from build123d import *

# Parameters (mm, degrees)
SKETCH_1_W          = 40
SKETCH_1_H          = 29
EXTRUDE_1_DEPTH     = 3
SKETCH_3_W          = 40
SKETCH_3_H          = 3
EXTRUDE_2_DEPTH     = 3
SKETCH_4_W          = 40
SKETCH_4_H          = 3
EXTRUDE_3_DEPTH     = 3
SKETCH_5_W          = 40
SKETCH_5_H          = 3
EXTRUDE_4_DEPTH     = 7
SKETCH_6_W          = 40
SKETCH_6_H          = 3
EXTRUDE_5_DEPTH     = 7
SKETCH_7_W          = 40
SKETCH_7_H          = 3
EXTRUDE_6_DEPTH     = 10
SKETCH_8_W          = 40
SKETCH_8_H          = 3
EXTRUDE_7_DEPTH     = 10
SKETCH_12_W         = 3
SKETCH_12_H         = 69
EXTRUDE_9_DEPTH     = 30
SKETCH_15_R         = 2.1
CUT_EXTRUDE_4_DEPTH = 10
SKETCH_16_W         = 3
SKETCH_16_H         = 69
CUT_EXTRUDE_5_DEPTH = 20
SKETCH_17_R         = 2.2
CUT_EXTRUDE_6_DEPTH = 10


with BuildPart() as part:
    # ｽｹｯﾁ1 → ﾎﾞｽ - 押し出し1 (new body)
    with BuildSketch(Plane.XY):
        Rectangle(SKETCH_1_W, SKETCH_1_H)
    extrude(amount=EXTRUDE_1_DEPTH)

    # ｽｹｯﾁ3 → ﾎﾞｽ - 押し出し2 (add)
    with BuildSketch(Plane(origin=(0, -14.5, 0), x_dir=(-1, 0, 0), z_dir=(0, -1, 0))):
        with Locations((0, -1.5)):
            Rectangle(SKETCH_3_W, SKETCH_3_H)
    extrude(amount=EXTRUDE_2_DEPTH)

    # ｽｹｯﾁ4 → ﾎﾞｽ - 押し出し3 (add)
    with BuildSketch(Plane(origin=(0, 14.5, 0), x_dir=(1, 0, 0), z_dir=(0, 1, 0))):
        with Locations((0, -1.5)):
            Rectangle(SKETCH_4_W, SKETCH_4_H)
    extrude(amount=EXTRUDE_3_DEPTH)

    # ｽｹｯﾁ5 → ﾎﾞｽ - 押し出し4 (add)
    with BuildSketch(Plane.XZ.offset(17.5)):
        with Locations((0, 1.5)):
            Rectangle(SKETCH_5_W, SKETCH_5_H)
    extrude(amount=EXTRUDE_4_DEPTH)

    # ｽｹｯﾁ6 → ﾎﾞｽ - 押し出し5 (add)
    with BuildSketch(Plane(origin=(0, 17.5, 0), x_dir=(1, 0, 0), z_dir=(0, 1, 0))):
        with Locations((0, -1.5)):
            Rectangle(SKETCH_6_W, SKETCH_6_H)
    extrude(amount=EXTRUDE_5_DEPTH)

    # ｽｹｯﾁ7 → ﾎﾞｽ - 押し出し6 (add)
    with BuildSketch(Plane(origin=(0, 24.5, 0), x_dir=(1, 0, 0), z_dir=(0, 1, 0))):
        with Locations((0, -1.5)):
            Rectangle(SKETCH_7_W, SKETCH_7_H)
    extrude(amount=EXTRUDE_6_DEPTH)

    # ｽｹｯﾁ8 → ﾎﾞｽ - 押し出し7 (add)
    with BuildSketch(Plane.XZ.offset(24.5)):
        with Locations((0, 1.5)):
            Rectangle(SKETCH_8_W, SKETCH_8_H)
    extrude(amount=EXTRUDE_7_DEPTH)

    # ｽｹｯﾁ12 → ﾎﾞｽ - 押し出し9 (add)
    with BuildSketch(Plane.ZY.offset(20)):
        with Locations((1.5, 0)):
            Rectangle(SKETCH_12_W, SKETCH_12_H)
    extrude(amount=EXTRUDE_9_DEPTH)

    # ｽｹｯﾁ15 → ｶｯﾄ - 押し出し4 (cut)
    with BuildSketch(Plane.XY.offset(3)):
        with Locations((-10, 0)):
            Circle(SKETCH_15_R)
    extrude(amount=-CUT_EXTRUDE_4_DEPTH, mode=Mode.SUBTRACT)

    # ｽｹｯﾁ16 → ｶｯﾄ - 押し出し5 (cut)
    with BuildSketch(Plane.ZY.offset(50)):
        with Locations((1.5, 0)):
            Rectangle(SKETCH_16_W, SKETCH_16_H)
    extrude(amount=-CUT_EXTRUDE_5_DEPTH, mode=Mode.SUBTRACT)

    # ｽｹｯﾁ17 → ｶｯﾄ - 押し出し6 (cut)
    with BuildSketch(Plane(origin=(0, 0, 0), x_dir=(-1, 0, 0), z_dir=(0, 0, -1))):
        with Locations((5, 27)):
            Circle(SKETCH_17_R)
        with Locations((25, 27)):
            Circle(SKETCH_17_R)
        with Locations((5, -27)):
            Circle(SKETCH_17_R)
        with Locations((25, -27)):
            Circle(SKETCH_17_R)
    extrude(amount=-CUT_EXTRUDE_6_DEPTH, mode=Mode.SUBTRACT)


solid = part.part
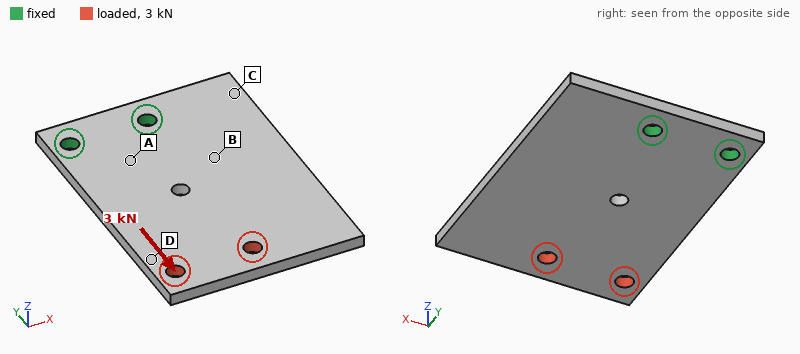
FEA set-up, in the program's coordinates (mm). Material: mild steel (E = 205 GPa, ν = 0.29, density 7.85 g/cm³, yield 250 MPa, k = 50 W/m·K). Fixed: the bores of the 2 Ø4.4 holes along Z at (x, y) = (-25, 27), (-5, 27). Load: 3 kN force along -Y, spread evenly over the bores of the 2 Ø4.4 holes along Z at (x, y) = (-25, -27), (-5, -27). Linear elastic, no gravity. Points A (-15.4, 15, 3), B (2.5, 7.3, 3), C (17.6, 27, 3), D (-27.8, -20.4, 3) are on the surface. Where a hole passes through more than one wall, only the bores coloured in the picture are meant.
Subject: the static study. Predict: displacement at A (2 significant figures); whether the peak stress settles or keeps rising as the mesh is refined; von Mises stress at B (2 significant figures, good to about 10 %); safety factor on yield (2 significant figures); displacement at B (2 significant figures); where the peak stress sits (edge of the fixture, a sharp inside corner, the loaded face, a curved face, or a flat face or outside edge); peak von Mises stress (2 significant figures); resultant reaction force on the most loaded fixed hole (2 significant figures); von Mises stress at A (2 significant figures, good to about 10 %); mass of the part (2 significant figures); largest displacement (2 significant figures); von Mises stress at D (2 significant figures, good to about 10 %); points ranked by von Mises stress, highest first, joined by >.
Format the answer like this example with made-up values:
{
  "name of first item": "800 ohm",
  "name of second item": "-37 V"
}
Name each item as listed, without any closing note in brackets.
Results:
{
  "displacement at A": "2.1 µm",
  "whether the peak stress settles or keeps rising as the mesh is refined": "settles",
  "von Mises stress at B": "15 MPa",
  "safety factor on yield": "2.5",
  "displacement at B": "2.3 µm",
  "where the peak stress sits": "the loaded face",
  "peak von Mises stress": "100 MPa",
  "resultant reaction force on the most loaded fixed hole": "1.5 kN",
  "von Mises stress at A": "26 MPa",
  "mass of the part": "79 g",
  "largest displacement": "13 µm",
  "von Mises stress at D": "45 MPa",
  "points ranked by von Mises stress, highest first, joined by >": "D > A > B > C"
}
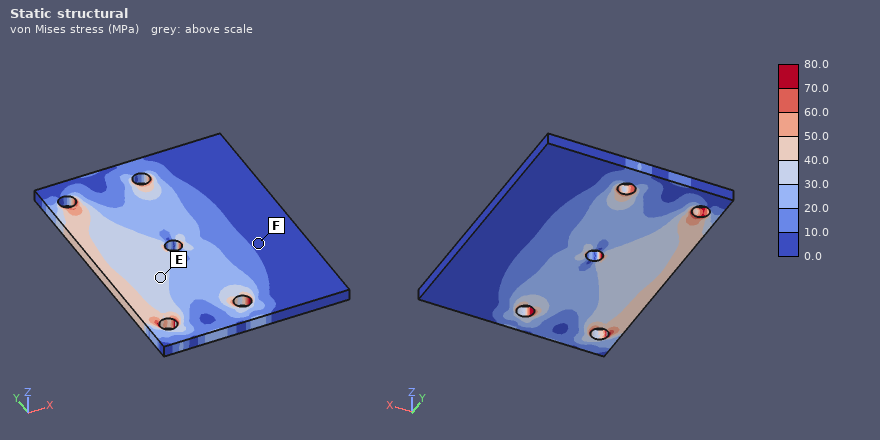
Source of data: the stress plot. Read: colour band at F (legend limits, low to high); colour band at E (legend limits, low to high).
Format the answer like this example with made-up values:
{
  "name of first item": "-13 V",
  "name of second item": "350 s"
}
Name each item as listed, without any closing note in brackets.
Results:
{
  "colour band at F": "0.0 to 10.0 MPa",
  "colour band at E": "30.0 to 40.0 MPa"
}
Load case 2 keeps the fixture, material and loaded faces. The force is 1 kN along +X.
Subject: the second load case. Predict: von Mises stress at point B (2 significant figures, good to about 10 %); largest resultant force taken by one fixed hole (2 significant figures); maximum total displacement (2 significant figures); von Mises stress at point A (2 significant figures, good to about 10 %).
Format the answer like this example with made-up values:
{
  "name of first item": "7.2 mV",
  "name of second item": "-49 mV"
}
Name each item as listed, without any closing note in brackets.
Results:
{
  "von Mises stress at point B": "21 MPa",
  "largest resultant force taken by one fixed hole": "2.4 kN",
  "maximum total displacement": "38 µm",
  "von Mises stress at point A": "39 MPa"
}
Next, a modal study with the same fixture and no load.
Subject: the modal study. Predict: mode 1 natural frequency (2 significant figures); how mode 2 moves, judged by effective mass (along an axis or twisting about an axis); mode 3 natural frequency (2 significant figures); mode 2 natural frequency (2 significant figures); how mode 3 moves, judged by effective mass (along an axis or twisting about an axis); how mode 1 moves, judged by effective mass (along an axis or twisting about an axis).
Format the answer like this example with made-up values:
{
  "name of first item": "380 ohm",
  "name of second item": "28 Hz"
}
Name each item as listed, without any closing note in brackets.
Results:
{
  "mode 1 natural frequency": "640 Hz",
  "how mode 2 moves, judged by effective mass": "twisting about Y",
  "mode 3 natural frequency": "3600 Hz",
  "mode 2 natural frequency": "1700 Hz",
  "how mode 3 moves, judged by effective mass": "along Z",
  "how mode 1 moves, judged by effective mass": "along Z"
}
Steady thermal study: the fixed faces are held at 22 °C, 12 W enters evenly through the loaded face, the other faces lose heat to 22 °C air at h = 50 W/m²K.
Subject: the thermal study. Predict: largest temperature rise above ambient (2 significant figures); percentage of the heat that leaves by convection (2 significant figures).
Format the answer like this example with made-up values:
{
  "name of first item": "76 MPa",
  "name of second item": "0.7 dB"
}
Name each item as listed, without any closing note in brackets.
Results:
{
  "largest temperature rise above ambient": "66 K",
  "percentage of the heat that leaves by convection": "67 %"
}
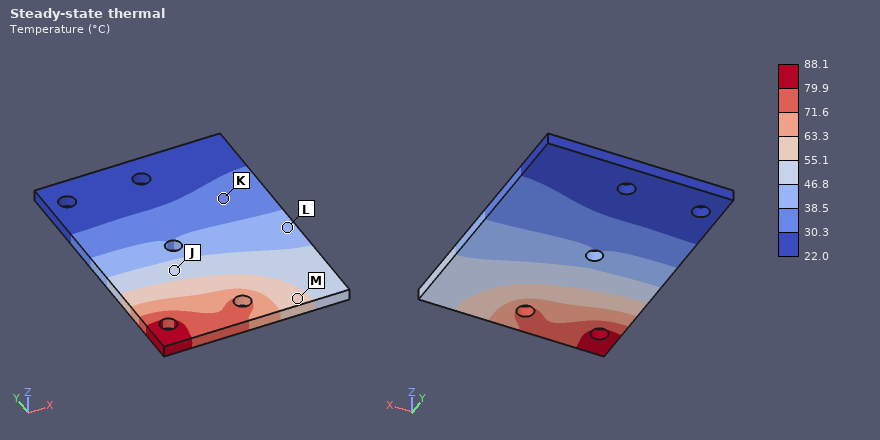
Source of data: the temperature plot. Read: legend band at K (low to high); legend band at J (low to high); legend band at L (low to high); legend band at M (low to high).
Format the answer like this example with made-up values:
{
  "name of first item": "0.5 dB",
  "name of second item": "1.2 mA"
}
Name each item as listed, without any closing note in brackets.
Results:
{
  "legend band at K": "30.3 to 38.5 °C",
  "legend band at J": "46.8 to 55.1 °C",
  "legend band at L": "38.5 to 46.8 °C",
  "legend band at M": "55.1 to 63.3 °C"
}
